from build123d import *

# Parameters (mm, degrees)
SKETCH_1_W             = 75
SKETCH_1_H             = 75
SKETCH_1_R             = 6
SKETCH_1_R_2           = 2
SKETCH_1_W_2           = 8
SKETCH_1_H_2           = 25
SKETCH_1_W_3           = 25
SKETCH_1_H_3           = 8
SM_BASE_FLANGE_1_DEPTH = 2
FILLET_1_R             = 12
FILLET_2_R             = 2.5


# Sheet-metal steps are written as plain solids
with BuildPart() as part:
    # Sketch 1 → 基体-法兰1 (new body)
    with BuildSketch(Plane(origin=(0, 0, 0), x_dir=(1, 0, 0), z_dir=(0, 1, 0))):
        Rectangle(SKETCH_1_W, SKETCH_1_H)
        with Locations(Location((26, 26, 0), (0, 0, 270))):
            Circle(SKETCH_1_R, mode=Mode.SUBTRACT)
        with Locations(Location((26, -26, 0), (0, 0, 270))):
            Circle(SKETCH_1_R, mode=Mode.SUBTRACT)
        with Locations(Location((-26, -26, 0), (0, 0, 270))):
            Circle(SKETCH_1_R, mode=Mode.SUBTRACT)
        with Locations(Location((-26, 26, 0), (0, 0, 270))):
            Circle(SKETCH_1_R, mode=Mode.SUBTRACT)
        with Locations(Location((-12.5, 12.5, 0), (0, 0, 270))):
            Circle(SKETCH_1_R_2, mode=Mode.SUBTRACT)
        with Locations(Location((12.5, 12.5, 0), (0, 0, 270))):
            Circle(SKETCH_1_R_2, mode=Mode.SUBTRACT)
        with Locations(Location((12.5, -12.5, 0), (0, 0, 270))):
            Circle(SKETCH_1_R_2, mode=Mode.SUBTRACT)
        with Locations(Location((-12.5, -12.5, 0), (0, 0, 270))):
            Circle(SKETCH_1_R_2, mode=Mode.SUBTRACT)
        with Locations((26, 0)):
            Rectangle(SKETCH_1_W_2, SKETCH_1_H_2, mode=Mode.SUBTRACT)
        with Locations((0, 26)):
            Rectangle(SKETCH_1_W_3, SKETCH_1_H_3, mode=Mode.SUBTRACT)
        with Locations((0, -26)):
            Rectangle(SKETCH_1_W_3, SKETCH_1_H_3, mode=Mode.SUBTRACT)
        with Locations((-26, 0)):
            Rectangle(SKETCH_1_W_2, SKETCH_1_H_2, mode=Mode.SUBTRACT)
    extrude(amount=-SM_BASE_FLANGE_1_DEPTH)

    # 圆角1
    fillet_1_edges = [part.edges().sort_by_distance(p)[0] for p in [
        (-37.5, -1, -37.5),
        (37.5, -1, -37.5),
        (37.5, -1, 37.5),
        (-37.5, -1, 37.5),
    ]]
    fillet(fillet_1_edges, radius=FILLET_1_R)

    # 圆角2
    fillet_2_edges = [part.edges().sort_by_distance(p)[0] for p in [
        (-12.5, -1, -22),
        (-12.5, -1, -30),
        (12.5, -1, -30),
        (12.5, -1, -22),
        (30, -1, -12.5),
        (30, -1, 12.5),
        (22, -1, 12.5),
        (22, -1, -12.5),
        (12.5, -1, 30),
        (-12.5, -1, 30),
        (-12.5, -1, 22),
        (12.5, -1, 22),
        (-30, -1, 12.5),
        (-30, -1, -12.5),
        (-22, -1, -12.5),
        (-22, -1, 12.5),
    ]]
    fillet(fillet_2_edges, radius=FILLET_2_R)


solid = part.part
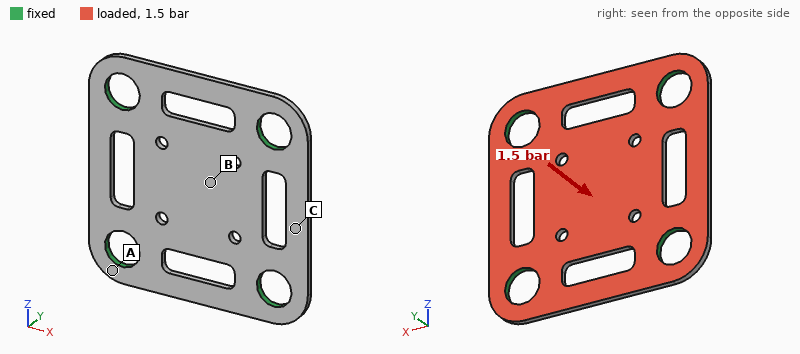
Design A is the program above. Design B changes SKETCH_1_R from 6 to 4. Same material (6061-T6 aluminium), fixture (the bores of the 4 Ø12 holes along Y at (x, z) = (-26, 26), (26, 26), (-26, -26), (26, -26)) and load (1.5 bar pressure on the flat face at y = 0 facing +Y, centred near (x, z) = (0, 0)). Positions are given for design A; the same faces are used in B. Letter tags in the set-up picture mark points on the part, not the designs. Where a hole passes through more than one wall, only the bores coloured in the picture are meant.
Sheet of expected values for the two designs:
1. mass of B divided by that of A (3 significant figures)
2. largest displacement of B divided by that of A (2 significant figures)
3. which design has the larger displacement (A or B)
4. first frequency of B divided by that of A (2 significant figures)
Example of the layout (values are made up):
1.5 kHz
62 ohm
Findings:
1.06
1.3
B
0.87
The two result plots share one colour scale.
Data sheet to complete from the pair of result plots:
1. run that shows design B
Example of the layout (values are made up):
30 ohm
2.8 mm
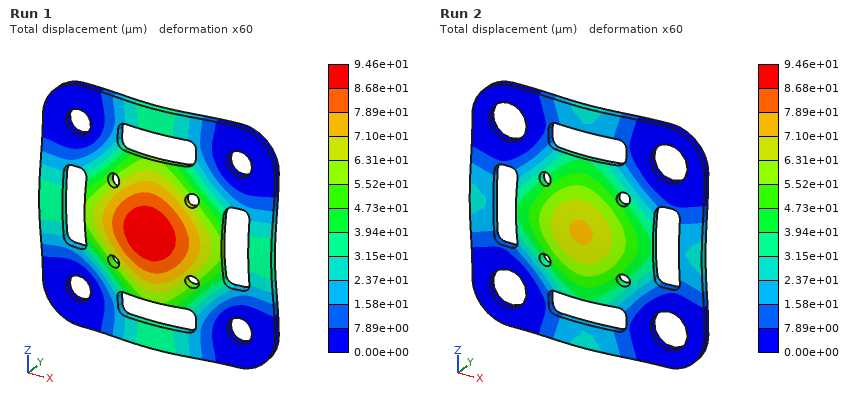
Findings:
Run 1
